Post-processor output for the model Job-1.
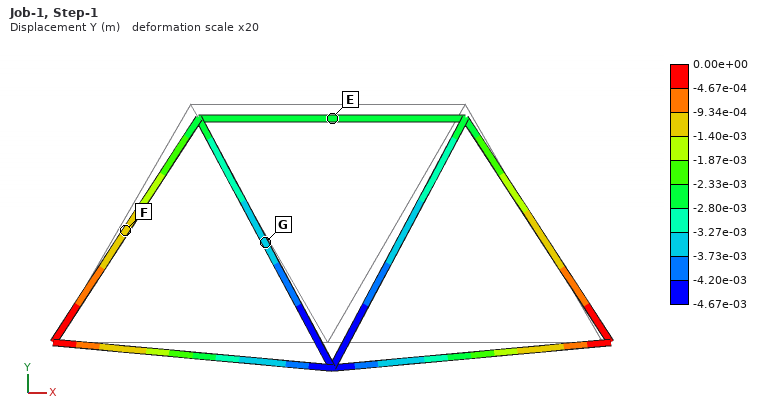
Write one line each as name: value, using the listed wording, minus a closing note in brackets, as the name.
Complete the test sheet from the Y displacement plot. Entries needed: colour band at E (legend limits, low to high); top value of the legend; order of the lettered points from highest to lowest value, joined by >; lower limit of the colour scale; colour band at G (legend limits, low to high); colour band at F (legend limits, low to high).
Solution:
colour band at E: -2.80e-03 to -2.33e-03 m
top value of the legend: 0.00e+00 m
order of the lettered points from highest to lowest value, joined by >: F > E > G
lower limit of the colour scale: -4.67e-03 m
colour band at G: -3.73e-03 to -3.27e-03 m
colour band at F: -1.40e-03 to -9.34e-04 m
